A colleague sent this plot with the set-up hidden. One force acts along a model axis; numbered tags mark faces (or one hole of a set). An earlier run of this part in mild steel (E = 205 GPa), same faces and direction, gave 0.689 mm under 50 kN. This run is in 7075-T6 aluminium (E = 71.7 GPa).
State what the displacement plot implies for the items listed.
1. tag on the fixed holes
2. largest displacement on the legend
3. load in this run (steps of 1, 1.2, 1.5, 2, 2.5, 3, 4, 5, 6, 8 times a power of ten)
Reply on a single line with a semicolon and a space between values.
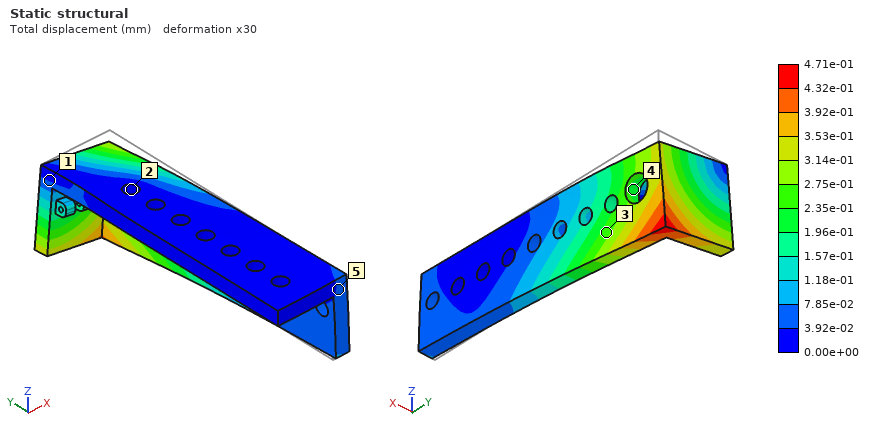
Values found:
2; 4.71e-01 mm; 12 kN
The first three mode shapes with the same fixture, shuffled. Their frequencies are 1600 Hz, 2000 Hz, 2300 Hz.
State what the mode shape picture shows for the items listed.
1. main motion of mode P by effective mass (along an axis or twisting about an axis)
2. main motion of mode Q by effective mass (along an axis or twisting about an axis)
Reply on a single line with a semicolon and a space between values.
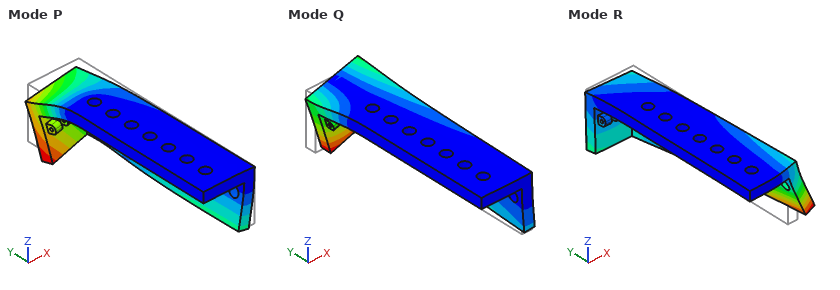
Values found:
along Z; along X
